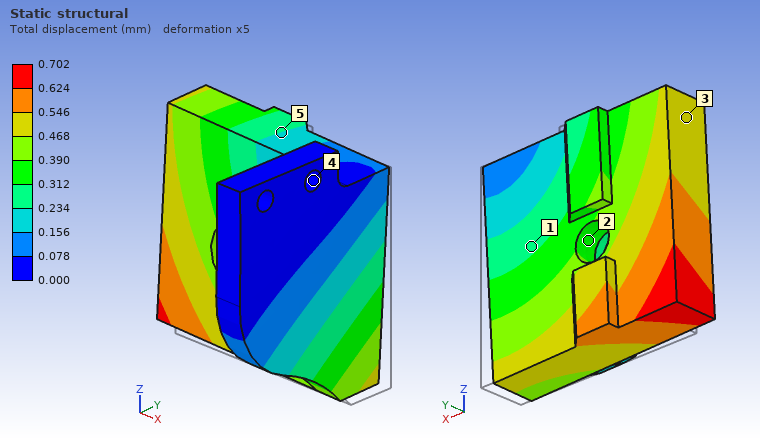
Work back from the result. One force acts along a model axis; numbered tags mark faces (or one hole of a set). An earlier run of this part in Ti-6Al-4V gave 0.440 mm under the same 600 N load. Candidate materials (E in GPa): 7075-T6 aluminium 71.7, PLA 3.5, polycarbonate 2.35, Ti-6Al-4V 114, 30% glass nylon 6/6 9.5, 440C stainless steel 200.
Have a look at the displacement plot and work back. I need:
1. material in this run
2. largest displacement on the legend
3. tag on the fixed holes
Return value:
7075-T6 aluminium
0.702 mm
4
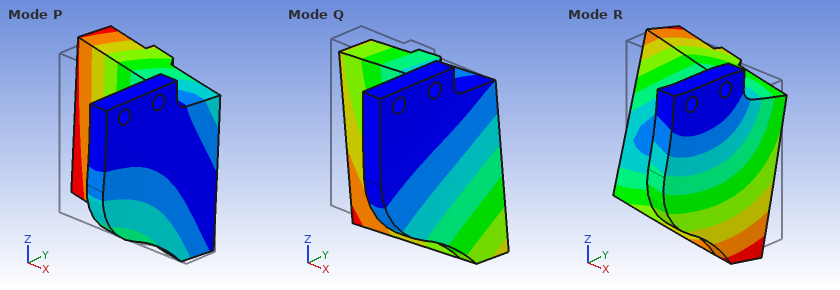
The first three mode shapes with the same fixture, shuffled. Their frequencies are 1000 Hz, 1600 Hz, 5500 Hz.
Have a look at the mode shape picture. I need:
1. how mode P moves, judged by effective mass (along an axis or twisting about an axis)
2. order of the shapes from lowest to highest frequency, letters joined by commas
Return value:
along Y
Q, P, R
